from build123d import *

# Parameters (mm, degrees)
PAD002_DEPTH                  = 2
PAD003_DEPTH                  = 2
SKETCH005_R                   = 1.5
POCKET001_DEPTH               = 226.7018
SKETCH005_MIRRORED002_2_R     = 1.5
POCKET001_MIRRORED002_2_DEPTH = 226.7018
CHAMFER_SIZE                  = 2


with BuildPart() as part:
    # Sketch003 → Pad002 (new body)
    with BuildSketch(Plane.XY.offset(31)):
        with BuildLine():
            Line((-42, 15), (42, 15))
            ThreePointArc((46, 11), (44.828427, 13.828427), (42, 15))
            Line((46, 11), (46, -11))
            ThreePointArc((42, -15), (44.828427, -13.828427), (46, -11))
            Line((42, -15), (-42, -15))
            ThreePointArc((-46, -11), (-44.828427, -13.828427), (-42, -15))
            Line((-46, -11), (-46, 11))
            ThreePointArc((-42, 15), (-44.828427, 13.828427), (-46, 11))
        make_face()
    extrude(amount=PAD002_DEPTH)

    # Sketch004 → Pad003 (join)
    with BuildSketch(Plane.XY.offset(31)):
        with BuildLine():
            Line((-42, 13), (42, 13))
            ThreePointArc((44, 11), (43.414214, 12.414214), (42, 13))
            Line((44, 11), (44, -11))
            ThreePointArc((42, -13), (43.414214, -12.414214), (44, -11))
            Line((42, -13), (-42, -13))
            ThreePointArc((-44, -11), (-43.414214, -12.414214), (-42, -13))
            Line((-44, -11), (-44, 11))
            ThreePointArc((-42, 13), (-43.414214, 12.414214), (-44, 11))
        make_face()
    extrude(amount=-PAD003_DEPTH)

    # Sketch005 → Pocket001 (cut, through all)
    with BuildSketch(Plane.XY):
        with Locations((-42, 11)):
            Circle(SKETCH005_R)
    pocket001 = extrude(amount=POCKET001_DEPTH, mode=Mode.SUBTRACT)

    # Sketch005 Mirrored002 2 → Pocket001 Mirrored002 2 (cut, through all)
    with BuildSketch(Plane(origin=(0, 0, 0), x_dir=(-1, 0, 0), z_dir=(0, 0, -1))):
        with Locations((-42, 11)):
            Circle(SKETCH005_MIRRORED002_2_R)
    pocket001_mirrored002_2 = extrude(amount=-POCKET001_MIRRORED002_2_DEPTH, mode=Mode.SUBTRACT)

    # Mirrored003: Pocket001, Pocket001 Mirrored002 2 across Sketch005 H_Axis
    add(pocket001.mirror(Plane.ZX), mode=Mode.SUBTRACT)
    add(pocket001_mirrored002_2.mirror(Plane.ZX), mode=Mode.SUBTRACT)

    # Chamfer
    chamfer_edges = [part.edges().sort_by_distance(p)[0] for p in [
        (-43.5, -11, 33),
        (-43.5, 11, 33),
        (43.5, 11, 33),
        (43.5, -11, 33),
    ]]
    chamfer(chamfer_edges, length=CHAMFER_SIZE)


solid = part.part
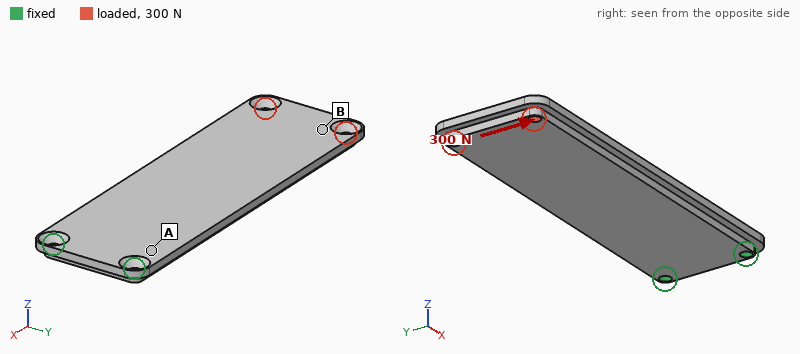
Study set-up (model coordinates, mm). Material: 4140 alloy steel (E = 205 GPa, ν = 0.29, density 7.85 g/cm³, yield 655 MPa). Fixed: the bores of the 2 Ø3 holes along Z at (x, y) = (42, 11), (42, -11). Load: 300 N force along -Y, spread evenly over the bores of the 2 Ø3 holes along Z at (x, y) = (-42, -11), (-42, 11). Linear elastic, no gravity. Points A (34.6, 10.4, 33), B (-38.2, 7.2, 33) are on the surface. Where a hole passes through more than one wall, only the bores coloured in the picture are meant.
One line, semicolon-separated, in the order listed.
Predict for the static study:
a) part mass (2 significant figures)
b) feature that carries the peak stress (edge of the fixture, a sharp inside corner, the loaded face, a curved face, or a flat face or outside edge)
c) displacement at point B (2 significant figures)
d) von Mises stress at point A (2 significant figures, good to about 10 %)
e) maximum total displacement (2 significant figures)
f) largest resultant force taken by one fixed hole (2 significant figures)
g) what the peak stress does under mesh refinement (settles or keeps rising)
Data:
77 g; edge of the fixture; 44 µm; 24 MPa; 54 µm; 1.1 kN; keeps rising
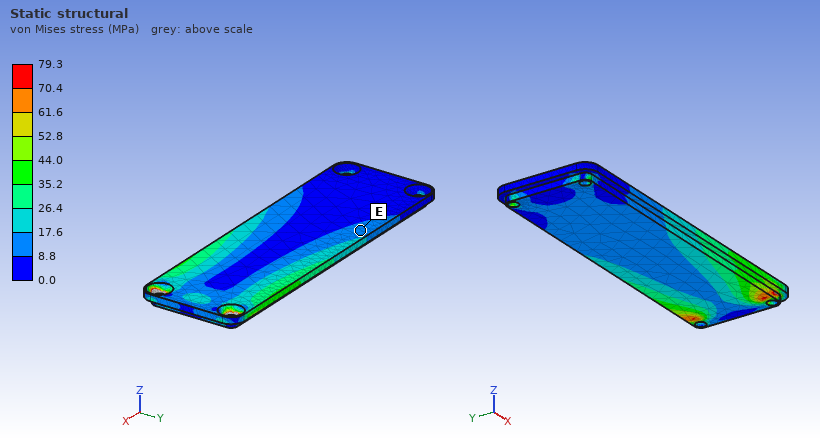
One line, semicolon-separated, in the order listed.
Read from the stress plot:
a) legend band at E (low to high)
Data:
8.8 to 17.6 MPa
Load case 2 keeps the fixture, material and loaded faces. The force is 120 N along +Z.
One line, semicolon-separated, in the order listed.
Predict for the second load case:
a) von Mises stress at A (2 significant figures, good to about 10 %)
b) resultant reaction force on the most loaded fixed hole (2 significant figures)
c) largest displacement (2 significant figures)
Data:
120 MPa; 130 N; 1.1 mm
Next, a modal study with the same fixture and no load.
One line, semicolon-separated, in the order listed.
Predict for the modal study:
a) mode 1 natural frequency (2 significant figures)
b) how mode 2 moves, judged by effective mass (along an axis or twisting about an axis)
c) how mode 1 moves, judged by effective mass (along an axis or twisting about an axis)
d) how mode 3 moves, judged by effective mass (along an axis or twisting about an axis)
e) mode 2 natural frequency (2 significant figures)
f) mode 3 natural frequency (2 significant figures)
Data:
370 Hz; along Z; along Z; along Y; 2400 Hz; 2600 Hz
